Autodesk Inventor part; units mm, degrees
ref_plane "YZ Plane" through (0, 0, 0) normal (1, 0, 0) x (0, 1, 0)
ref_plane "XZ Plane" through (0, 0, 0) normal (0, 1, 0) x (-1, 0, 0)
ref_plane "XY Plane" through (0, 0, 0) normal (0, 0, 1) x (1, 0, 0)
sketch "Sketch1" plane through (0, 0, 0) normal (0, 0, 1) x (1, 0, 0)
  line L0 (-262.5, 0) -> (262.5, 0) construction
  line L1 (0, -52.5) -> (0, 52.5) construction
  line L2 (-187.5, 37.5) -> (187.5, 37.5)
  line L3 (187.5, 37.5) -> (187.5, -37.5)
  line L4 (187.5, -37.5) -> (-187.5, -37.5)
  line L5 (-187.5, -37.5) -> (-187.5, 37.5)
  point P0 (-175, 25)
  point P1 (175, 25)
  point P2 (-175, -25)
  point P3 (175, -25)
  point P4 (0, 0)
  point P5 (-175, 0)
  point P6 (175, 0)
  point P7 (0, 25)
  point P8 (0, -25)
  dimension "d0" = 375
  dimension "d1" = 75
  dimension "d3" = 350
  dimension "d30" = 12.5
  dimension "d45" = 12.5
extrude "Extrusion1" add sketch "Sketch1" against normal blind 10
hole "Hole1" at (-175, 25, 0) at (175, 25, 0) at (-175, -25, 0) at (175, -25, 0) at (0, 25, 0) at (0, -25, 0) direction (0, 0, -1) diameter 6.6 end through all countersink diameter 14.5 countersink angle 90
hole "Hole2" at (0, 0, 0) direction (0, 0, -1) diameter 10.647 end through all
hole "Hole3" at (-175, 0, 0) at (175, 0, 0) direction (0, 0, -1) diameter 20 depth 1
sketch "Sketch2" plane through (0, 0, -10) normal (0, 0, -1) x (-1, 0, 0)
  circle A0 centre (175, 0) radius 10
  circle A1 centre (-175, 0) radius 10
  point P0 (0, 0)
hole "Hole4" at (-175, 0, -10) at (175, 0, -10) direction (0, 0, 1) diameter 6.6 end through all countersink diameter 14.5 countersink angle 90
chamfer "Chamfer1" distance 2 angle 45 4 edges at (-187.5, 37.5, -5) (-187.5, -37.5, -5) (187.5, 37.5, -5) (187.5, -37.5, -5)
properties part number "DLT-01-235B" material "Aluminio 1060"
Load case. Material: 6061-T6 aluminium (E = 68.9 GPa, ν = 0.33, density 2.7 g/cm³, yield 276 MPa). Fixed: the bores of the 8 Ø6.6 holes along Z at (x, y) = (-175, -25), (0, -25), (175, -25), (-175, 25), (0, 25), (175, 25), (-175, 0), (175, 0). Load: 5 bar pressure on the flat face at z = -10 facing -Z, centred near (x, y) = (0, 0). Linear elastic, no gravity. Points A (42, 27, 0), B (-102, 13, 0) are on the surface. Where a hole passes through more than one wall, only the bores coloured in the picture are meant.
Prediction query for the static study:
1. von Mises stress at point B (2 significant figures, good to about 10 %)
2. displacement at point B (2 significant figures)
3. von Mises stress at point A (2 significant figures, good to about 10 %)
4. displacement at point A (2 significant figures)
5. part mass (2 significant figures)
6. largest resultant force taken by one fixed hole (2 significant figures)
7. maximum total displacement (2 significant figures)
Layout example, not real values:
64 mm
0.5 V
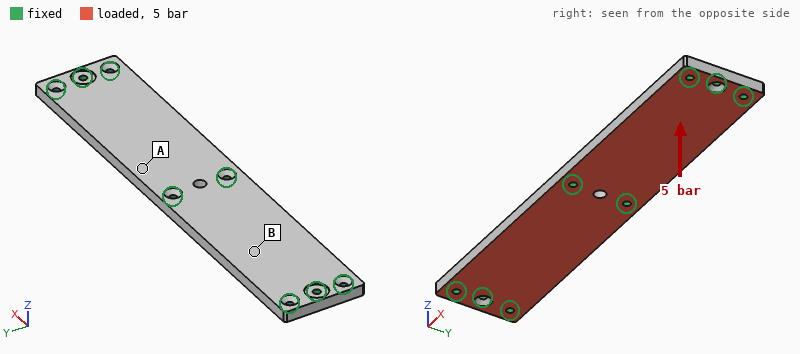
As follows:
38 MPa
0.23 mm
14 MPa
0.14 mm
740 g
3.4 kN
0.26 mm
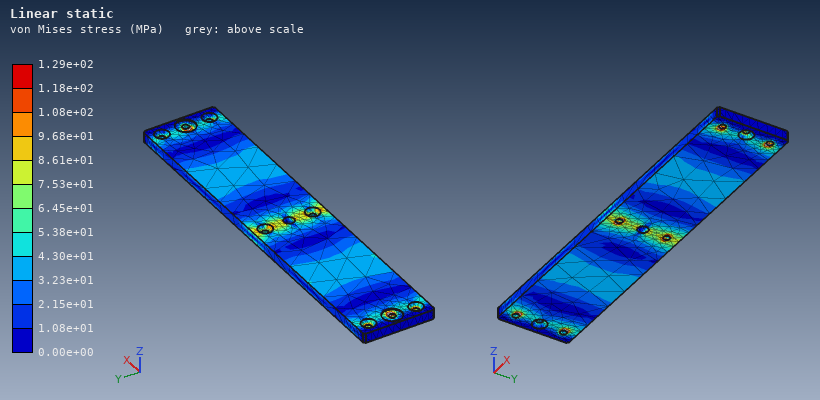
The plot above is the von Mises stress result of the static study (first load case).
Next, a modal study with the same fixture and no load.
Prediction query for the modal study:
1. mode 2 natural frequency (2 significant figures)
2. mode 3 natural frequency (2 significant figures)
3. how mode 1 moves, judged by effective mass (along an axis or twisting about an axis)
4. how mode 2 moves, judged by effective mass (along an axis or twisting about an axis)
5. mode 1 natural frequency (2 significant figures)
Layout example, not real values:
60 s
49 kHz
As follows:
1600 Hz
2700 Hz
twisting about Y
along Z
1400 Hz
